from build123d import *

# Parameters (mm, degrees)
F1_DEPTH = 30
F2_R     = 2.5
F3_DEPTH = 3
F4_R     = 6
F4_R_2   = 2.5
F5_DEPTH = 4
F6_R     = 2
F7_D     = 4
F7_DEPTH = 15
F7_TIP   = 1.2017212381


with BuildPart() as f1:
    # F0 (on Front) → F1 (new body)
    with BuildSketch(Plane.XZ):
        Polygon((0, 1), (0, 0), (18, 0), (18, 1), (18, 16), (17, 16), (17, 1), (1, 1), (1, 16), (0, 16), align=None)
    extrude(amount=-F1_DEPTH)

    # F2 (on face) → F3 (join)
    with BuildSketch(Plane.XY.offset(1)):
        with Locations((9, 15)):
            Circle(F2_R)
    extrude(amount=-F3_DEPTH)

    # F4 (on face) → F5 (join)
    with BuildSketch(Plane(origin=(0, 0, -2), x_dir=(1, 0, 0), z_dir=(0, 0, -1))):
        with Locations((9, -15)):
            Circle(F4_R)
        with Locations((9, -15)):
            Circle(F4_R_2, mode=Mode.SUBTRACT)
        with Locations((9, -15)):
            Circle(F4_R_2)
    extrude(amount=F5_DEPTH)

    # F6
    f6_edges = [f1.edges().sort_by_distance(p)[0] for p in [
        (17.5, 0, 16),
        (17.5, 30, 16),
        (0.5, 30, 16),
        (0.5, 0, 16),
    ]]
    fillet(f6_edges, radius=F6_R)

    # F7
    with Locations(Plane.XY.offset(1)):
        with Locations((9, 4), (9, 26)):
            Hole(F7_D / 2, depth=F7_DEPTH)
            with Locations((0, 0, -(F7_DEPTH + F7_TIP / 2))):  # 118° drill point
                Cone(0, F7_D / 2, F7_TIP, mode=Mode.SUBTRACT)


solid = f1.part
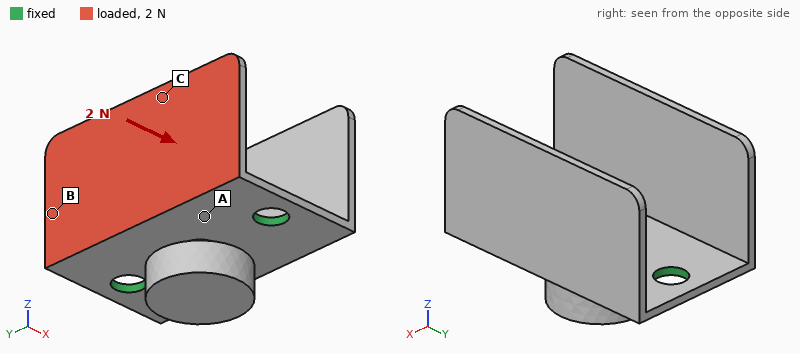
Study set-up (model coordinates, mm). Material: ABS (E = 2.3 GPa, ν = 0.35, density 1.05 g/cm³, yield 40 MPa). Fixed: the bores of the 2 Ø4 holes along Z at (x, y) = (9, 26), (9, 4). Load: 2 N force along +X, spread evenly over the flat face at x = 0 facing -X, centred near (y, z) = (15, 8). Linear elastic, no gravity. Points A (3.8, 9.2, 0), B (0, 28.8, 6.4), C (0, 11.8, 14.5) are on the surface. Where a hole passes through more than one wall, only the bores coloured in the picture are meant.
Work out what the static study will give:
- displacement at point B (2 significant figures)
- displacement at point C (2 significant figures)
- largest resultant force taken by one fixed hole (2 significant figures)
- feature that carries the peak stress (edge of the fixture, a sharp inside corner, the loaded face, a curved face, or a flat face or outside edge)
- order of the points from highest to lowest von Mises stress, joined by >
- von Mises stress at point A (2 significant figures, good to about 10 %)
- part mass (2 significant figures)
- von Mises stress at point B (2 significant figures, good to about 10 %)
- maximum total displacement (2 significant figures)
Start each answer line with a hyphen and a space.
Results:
- 0.15 mm
- 0.36 mm
- 1.0 N
- a flat face or outside edge
- A > B > C
- 2.5 MPa
- 2.0 g
- 1.1 MPa
- 0.40 mm
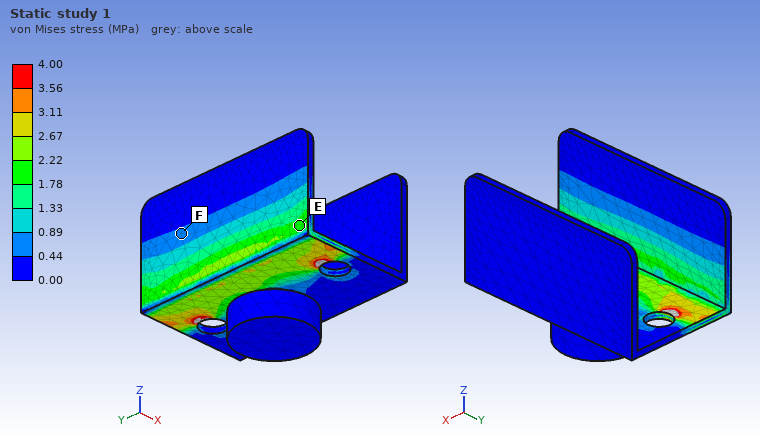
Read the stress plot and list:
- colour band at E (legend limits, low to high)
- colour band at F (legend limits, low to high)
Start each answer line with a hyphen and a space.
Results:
- 1.78 to 2.22 MPa
- 0.44 to 0.89 MPa
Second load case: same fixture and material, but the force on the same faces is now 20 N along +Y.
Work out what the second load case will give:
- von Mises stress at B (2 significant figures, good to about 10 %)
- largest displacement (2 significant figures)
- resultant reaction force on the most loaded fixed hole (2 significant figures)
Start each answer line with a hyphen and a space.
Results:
- 2.8 MPa
- 0.49 mm
- 14 N
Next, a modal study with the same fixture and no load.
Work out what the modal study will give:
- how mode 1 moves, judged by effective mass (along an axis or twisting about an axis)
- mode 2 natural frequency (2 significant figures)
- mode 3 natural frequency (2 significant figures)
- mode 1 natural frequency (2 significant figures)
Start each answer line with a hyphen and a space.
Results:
- along X
- 610 Hz
- 1100 Hz
- 580 Hz
